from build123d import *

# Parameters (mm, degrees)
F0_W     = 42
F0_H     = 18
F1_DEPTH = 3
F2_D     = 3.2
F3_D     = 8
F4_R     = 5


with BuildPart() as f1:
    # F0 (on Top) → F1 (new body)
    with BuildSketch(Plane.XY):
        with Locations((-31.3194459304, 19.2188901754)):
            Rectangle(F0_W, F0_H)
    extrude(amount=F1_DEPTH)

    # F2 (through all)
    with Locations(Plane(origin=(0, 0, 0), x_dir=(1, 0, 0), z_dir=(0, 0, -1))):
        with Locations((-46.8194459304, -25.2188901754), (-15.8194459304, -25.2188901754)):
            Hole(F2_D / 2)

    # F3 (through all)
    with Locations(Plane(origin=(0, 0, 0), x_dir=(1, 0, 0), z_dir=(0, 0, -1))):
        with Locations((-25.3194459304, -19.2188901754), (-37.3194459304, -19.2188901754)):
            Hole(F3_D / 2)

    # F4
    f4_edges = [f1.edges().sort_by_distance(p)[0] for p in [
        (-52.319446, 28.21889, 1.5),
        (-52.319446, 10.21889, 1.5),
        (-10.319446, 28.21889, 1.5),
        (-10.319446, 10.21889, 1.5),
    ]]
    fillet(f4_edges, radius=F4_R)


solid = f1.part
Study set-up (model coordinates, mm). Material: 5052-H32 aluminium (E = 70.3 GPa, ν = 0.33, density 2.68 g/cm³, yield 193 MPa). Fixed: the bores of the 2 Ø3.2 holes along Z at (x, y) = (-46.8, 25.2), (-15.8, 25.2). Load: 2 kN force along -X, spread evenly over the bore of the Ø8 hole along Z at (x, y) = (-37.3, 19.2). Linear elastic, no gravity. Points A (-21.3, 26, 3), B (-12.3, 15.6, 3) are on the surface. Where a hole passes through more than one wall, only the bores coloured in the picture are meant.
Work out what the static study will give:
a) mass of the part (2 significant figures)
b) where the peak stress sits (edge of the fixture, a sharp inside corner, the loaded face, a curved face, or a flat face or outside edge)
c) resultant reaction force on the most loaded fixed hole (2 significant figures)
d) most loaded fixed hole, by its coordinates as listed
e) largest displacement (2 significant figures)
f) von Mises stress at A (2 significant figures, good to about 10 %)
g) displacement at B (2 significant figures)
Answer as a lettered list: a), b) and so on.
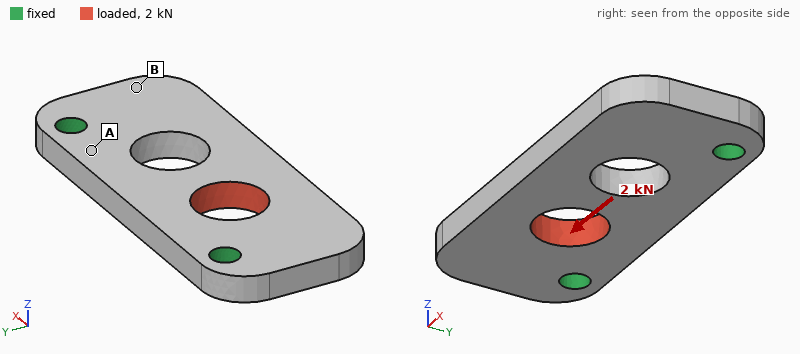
a) 5.0 g
b) edge of the fixture
c) 1.3 kN
d) (-46.8, 25.2)
e) 18 µm
f) 40 MPa
g) 8.8 µm
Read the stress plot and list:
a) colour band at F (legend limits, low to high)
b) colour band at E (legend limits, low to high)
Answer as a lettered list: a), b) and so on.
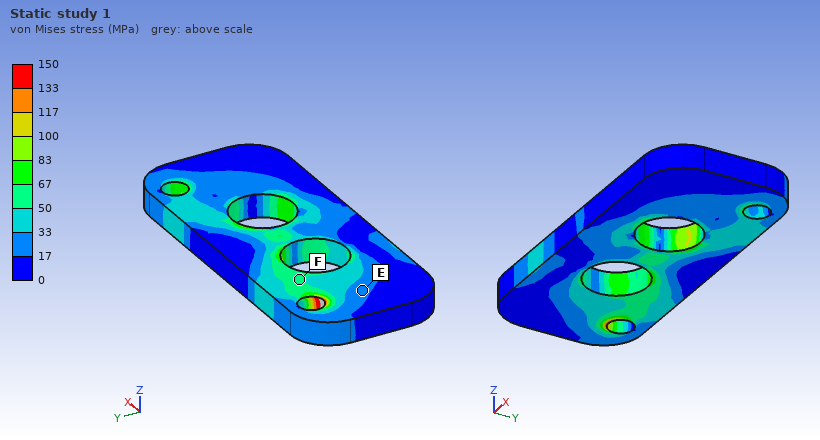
a) 50 to 67 MPa
b) 17 to 33 MPa
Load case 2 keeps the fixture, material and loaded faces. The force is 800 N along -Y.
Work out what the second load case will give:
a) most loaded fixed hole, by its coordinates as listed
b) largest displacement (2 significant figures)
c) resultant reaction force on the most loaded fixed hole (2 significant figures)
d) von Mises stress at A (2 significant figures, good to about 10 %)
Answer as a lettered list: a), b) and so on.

a) (-46.8, 25.2)
b) 9.6 µm
c) 590 N
d) 10 MPa
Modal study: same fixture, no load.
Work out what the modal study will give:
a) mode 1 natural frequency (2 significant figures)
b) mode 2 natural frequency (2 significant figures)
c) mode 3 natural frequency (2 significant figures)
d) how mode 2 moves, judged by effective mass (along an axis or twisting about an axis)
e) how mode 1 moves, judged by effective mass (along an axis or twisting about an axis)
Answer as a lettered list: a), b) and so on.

a) 8200 Hz
b) 14 kHz
c) 17 kHz
d) twisting about Y
e) along Z
